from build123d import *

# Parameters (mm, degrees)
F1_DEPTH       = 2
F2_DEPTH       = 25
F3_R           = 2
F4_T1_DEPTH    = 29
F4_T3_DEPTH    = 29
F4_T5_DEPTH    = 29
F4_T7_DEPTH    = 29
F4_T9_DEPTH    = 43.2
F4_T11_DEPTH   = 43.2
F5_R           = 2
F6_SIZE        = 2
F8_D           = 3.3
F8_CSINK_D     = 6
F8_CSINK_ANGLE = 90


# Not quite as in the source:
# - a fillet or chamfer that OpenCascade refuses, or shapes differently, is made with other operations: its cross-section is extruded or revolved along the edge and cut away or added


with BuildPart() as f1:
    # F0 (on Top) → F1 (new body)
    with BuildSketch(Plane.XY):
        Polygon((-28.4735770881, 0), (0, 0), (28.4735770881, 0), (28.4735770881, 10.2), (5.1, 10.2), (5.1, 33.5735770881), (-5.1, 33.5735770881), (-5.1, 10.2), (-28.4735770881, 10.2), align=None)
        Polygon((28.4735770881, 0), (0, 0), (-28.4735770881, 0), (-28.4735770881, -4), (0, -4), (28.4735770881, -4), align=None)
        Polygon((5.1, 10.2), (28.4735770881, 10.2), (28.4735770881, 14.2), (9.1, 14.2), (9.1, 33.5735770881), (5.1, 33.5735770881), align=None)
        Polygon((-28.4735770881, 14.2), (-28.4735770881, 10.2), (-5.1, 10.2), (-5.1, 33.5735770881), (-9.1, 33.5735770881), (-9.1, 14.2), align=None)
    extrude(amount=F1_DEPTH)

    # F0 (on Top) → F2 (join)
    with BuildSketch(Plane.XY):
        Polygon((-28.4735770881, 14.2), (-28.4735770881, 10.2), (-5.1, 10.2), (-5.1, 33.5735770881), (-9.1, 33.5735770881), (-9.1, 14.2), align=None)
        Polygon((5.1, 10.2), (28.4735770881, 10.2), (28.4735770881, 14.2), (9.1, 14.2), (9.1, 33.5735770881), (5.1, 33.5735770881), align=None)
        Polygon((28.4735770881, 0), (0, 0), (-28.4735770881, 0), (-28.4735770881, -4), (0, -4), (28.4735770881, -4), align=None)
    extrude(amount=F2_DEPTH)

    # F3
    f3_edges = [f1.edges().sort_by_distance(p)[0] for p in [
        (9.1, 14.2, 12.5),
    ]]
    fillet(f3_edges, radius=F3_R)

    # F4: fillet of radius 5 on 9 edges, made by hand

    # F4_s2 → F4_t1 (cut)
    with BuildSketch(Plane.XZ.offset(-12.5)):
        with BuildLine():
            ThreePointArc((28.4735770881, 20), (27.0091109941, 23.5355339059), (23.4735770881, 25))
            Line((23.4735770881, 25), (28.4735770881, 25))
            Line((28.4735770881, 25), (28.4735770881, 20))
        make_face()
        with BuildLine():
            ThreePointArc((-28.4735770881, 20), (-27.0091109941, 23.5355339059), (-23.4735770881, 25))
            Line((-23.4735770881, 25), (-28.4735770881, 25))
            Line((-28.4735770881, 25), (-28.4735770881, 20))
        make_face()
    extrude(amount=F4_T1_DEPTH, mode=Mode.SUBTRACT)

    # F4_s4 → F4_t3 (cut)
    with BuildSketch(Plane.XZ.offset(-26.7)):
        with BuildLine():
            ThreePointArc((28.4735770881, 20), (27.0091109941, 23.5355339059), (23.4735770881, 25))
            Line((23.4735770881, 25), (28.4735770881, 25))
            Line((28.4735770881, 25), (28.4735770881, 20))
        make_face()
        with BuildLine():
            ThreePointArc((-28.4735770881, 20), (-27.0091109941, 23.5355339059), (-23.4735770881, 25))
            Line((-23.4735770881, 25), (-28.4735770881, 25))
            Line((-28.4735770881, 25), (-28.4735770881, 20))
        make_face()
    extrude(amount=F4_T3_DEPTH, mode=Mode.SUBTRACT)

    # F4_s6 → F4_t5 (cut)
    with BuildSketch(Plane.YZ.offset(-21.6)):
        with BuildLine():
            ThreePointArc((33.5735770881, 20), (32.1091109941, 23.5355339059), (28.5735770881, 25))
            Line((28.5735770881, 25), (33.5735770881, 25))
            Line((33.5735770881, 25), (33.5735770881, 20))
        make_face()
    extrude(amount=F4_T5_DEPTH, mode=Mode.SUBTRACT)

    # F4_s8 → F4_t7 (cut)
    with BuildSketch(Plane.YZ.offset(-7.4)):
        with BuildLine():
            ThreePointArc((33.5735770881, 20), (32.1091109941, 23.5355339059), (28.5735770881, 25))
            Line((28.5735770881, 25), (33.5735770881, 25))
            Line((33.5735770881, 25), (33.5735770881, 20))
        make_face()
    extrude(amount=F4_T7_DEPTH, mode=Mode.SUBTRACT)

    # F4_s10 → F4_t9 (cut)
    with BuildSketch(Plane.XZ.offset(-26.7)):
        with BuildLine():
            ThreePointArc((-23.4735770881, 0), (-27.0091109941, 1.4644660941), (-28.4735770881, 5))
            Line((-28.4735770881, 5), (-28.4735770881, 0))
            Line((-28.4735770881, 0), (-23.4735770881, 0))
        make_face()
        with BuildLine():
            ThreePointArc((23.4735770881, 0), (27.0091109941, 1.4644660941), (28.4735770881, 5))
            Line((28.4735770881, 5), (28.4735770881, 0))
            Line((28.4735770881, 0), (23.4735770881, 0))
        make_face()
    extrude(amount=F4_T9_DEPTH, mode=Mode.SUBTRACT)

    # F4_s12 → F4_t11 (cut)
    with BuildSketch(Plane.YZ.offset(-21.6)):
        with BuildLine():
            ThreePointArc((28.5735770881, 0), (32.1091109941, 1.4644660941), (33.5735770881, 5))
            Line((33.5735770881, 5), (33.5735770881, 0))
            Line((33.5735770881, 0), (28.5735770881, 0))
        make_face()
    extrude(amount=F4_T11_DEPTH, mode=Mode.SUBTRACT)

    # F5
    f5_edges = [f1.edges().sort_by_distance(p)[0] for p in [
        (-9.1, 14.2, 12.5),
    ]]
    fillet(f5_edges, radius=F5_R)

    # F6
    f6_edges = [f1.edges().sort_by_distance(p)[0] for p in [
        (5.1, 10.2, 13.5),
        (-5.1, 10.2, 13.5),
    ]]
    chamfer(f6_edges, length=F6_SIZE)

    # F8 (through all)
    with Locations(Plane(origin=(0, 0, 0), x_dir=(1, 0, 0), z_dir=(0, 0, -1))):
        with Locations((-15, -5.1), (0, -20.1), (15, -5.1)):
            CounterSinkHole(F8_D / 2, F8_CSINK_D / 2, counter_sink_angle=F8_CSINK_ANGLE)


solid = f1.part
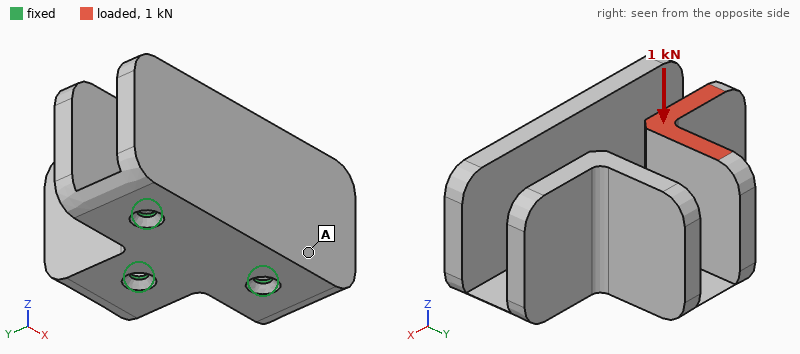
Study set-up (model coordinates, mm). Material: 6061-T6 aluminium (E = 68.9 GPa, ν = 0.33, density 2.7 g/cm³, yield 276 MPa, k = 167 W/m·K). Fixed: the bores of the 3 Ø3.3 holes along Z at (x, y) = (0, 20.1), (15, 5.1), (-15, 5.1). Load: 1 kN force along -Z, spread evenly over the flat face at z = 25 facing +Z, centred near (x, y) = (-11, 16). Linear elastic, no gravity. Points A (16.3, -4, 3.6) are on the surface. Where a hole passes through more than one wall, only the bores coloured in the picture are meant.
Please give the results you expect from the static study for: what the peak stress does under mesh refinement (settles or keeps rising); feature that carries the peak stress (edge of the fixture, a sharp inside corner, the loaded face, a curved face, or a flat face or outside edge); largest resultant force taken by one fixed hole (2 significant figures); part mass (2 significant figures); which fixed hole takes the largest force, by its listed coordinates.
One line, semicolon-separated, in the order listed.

keeps rising; edge of the fixture; 620 N; 41 g; (0, 20.1)
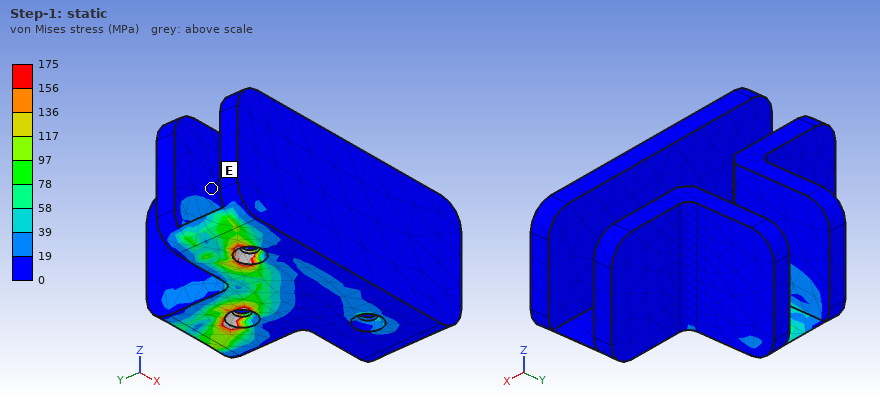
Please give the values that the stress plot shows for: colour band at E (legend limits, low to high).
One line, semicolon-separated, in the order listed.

0 to 19 MPa
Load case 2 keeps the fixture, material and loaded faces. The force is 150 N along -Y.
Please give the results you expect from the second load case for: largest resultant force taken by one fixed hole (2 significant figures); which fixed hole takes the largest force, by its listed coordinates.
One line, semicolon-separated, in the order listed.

250 N; (0, 20.1)
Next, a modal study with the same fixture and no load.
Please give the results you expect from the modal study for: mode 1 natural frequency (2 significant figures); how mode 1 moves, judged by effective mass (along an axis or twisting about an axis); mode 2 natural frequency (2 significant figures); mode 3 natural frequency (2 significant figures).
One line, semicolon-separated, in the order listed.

1500 Hz; along Y; 2100 Hz; 2400 Hz
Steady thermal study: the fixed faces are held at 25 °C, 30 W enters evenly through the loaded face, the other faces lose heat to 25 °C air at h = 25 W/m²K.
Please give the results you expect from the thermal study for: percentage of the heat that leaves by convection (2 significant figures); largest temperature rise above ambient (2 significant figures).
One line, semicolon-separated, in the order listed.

9.4 %; 47 K
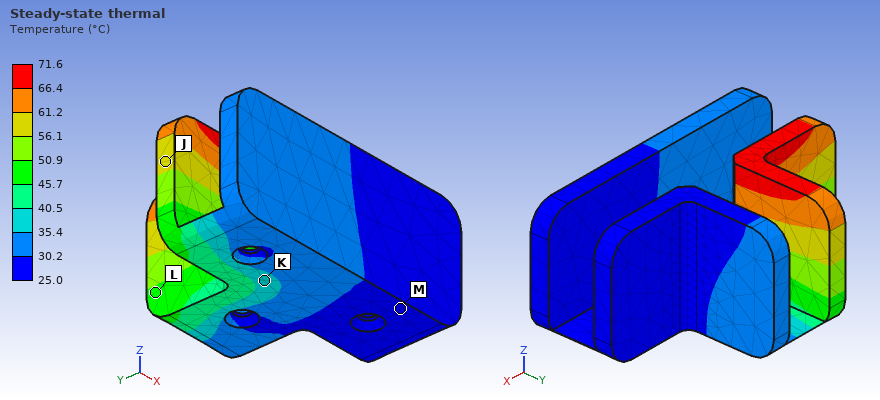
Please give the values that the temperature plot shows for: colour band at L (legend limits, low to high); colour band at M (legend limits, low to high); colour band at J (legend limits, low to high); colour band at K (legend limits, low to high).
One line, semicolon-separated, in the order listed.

45.7 to 50.9 °C; 25.0 to 30.2 °C; 56.1 to 61.2 °C; 35.4 to 40.5 °C
